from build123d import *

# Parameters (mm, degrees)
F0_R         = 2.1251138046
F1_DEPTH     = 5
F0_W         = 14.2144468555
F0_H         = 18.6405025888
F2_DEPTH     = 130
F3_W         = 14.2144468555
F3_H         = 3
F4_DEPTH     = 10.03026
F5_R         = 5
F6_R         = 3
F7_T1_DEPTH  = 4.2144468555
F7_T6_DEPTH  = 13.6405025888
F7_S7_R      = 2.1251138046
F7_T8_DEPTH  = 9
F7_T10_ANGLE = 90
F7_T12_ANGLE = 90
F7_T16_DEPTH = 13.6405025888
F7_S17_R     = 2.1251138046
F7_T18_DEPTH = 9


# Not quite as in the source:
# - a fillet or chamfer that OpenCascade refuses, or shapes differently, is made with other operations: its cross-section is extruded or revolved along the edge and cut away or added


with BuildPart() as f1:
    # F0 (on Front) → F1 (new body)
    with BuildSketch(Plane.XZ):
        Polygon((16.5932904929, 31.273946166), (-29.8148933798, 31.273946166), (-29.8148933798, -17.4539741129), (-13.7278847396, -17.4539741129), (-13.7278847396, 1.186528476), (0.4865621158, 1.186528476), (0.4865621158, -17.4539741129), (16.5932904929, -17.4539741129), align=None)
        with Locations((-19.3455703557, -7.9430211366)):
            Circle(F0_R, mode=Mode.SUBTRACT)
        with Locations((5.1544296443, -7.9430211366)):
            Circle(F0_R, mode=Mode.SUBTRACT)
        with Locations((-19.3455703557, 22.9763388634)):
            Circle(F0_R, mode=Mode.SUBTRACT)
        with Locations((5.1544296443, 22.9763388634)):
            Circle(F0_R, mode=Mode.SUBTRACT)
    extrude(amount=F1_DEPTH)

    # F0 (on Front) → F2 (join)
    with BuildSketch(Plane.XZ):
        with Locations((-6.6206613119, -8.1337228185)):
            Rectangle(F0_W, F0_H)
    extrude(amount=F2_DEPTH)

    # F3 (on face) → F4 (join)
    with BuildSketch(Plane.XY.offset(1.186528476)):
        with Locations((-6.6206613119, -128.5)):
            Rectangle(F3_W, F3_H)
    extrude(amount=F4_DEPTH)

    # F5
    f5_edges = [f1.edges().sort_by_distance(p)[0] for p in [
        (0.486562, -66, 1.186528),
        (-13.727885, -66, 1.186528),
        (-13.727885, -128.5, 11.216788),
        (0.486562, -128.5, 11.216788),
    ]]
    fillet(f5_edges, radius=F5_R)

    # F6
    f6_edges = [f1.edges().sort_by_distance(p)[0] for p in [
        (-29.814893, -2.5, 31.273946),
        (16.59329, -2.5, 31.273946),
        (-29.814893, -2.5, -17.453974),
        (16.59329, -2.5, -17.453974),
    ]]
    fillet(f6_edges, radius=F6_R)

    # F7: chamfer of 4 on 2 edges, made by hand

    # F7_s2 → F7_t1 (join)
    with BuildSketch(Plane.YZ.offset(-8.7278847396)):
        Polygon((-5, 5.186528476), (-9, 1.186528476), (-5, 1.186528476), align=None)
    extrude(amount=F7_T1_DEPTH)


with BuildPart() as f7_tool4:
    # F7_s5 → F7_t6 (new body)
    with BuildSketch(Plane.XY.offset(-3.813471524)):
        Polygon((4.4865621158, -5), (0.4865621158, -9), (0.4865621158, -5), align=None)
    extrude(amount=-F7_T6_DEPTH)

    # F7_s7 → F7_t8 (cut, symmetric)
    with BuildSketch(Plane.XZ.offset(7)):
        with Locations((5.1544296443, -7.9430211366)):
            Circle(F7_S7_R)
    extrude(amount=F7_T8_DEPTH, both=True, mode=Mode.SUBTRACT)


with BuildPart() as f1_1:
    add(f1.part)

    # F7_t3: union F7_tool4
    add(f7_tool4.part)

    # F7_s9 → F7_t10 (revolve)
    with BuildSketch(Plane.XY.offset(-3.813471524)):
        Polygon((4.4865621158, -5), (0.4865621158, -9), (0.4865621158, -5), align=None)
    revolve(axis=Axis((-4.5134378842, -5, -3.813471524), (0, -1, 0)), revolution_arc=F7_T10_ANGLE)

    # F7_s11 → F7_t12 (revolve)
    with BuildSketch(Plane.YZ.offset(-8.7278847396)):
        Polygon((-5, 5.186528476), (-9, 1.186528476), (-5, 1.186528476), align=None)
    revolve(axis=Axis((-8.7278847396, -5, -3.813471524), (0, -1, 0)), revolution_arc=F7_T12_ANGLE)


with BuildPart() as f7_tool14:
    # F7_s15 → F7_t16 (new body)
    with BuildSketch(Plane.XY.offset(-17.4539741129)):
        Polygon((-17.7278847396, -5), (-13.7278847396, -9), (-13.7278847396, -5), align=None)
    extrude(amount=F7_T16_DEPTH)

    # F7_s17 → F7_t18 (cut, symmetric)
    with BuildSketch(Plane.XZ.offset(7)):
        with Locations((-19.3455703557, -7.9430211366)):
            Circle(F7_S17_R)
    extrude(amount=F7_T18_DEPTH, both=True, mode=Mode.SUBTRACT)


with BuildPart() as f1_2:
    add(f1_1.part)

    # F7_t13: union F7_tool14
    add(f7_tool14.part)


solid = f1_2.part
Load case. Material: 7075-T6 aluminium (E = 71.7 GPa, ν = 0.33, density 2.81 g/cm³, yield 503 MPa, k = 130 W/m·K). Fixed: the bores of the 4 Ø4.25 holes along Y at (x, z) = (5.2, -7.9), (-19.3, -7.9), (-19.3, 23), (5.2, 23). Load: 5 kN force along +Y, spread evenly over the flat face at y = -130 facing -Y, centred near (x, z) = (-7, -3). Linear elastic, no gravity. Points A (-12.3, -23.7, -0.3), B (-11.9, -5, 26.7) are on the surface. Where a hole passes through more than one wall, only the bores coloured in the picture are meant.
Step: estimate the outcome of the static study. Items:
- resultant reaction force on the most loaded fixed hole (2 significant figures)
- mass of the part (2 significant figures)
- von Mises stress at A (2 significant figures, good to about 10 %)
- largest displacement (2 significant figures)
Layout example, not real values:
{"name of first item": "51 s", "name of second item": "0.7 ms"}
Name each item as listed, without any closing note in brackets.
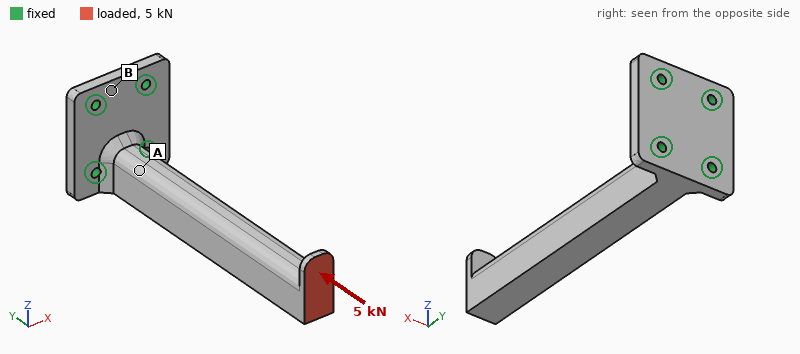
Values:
{"resultant reaction force on the most loaded fixed hole": "2.5 kN", "mass of the part": "120 g", "von Mises stress at A": "49 MPa", "largest displacement": "0.63 mm"}
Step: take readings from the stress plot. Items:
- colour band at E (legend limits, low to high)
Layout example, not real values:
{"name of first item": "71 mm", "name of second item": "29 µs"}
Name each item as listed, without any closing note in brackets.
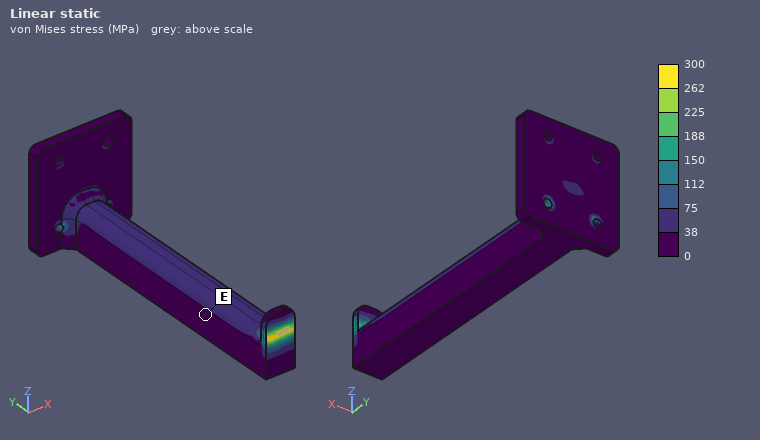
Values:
{"colour band at E": "0 to 38 MPa"}
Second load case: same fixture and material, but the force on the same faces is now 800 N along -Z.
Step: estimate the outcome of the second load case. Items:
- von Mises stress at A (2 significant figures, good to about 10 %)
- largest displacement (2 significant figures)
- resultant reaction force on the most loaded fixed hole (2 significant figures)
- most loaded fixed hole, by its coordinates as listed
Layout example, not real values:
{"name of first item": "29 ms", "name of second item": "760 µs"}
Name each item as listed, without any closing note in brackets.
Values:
{"von Mises stress at A": "100 MPa", "largest displacement": "1.7 mm", "resultant reaction force on the most loaded fixed hole": "1.4 kN", "most loaded fixed hole, by its coordinates as listed": "(5.2, -7.9)"}
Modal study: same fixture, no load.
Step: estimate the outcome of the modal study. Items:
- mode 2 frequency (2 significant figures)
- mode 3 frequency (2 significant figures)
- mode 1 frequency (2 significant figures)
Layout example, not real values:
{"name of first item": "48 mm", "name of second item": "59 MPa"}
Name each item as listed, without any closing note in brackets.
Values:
{"mode 2 frequency": "680 Hz", "mode 3 frequency": "4000 Hz", "mode 1 frequency": "670 Hz"}
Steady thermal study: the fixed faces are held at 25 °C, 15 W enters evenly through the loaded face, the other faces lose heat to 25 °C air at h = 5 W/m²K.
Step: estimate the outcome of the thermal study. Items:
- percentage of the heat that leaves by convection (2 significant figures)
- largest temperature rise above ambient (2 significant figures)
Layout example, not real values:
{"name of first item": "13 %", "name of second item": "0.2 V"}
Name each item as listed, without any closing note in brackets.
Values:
{"percentage of the heat that leaves by convection": "8.0 %", "largest temperature rise above ambient": "63 K"}
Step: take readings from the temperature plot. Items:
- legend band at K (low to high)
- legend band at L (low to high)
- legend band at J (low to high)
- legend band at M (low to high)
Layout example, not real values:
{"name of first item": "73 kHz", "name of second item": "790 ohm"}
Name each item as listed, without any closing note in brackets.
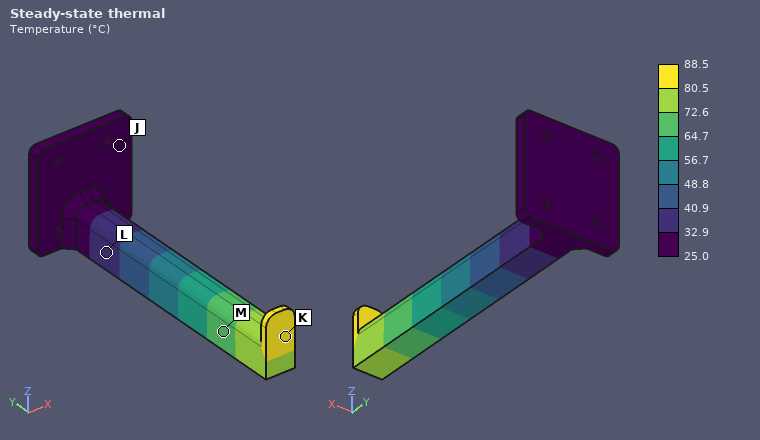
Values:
{"legend band at K": "80.5 to 88.5 °C", "legend band at L": "32.9 to 40.9 °C", "legend band at J": "25.0 to 32.9 °C", "legend band at M": "64.7 to 72.6 °C"}
